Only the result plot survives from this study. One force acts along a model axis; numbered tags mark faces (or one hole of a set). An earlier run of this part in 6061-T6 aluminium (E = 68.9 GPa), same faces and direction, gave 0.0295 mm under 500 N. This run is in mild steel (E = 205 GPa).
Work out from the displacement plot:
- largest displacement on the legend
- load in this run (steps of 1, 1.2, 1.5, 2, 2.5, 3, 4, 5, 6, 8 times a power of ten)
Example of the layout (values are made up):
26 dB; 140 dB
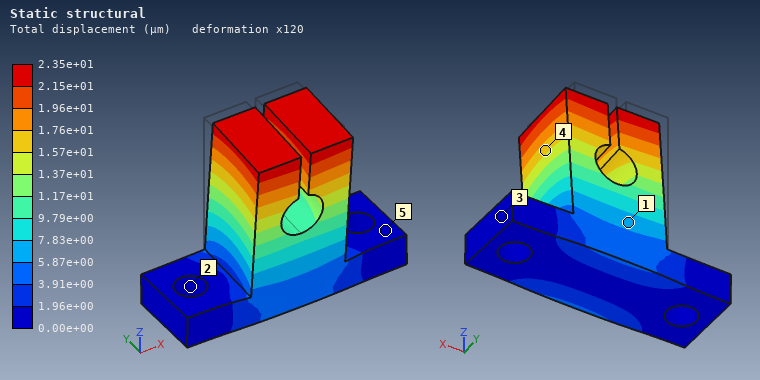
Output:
2.35e+01 µm; 1.2 kN
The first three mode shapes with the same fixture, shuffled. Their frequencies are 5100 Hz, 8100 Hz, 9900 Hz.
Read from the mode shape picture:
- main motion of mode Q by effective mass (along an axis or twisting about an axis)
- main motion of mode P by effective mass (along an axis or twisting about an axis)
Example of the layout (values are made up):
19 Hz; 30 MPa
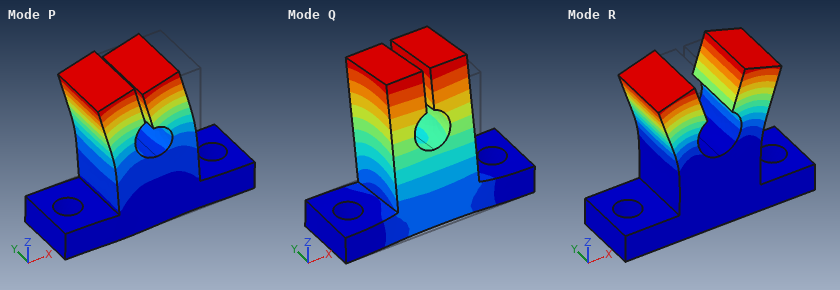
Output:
along Y; along X
